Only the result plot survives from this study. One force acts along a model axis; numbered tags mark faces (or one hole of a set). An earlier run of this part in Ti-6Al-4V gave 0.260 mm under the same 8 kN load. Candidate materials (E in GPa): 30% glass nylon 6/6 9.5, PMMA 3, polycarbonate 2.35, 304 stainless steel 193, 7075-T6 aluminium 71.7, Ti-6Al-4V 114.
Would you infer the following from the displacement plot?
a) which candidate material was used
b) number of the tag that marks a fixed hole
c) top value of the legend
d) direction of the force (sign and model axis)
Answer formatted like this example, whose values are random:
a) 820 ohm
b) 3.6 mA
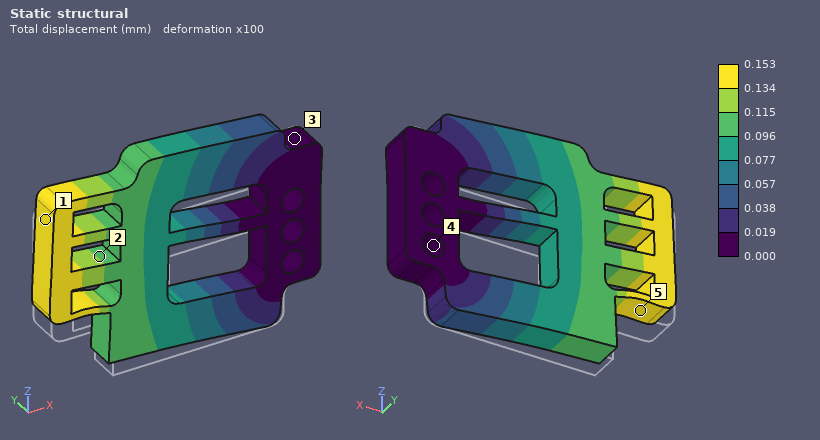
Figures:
a) 304 stainless steel
b) 4
c) 0.153 mm
d) +Z
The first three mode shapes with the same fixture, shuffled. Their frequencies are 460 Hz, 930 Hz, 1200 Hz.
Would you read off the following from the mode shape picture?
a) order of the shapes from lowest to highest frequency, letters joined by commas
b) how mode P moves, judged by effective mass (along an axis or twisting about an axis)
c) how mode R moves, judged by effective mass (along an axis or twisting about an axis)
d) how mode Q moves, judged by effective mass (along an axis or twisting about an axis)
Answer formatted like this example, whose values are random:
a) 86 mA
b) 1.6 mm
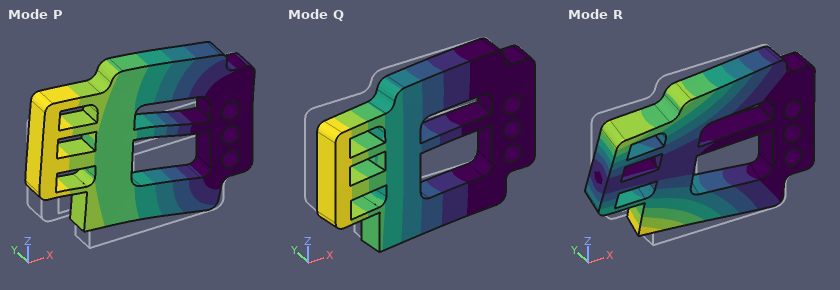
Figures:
a) Q, P, R
b) along Z
c) twisting about X
d) along Y
